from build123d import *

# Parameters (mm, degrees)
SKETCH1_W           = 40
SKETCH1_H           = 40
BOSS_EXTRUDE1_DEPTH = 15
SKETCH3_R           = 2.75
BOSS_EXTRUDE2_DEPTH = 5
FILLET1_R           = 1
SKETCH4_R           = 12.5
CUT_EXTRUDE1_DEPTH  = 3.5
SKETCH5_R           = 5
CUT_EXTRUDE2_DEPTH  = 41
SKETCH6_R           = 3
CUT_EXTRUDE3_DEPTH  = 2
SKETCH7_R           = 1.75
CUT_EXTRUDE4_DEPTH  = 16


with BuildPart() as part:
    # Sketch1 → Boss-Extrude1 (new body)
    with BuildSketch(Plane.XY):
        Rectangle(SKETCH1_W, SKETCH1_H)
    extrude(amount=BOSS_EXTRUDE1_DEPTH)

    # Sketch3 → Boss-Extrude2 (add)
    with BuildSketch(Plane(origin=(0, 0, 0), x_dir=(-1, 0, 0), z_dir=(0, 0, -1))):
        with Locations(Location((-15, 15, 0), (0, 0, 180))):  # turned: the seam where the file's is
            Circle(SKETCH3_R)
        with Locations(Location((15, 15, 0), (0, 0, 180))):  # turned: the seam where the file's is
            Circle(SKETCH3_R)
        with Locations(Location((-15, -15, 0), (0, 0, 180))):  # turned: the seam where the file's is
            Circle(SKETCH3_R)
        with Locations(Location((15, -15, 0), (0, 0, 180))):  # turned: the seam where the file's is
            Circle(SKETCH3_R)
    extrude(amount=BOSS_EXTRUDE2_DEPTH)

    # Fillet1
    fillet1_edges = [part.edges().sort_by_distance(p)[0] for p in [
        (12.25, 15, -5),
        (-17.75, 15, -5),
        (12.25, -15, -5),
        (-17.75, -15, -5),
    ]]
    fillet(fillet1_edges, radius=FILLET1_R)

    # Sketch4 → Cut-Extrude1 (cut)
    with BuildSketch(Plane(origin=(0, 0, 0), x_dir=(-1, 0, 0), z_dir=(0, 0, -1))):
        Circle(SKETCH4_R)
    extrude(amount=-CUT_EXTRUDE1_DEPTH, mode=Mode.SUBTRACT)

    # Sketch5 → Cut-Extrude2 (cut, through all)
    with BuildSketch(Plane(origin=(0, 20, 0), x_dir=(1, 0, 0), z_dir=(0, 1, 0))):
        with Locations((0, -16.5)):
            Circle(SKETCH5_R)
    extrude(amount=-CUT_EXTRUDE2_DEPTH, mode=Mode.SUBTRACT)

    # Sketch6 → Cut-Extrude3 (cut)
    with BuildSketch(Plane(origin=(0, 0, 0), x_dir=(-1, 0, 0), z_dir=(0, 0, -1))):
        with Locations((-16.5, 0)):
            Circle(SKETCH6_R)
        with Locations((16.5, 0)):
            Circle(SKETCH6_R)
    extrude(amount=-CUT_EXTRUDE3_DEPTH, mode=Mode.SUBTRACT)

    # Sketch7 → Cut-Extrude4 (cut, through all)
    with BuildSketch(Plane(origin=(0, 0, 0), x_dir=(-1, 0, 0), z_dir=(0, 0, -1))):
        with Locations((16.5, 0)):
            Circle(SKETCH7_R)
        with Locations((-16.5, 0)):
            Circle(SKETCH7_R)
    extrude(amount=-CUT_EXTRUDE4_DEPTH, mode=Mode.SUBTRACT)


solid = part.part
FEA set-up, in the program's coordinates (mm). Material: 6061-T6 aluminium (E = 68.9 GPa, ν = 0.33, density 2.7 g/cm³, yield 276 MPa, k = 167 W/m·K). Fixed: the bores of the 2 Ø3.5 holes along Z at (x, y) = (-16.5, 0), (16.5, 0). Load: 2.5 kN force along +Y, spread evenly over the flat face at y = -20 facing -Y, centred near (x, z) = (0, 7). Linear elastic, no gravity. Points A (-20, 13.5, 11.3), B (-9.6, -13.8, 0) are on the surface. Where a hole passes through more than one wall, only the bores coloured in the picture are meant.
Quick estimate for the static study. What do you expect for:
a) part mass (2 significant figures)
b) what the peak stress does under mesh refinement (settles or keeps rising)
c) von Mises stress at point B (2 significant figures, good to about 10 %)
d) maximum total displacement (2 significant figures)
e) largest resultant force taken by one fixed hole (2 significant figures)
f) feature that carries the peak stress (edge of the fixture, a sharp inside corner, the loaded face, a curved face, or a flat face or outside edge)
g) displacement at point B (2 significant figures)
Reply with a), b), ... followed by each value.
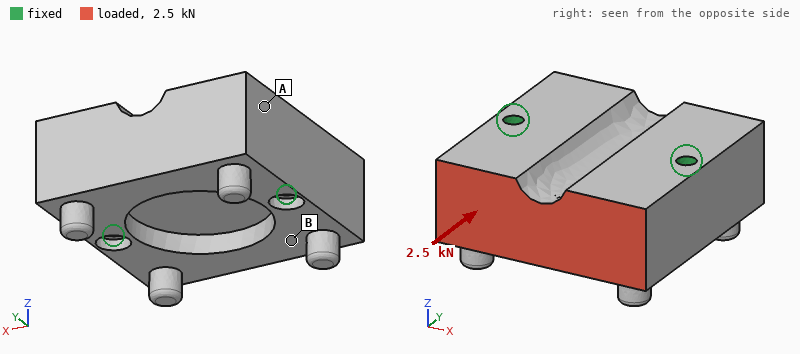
a) 58 g
b) keeps rising
c) 5.9 MPa
d) 3.7 µm
e) 1.3 kN
f) edge of the fixture
g) 2.5 µm
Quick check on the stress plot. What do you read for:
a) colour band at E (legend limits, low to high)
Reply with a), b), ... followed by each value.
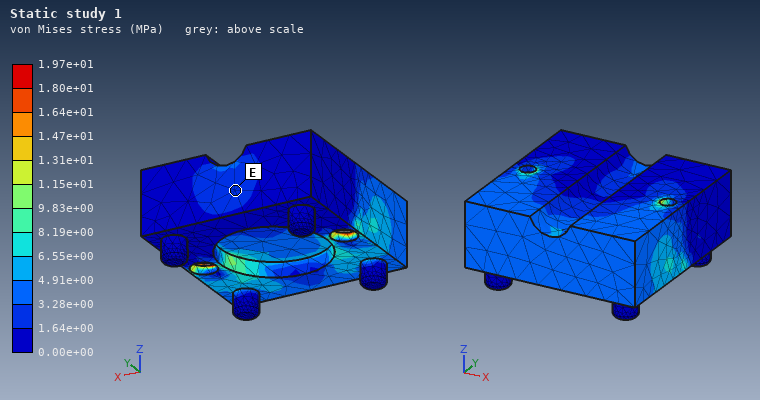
a) 1.64e+00 to 3.28e+00 MPa
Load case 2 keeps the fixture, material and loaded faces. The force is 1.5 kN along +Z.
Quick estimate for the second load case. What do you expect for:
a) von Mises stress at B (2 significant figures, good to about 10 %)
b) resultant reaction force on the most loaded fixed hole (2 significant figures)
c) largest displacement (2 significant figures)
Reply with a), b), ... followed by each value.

a) 9.0 MPa
b) 750 N
c) 19 µm
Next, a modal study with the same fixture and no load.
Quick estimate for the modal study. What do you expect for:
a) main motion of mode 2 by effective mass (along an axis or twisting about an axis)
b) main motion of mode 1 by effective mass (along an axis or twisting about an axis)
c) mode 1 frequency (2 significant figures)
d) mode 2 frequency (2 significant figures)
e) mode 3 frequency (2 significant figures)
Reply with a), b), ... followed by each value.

a) along Z
b) twisting about X
c) 14 kHz
d) 17 kHz
e) 22 kHz
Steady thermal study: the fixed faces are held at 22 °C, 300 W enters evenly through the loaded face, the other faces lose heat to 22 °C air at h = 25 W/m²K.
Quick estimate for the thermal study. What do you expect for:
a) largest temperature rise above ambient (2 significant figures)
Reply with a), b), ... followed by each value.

a) 83 K
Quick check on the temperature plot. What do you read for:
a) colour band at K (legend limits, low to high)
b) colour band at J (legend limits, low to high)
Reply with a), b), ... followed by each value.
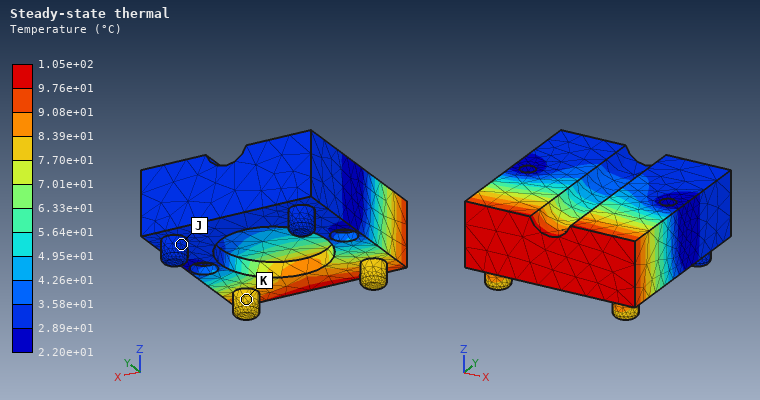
a) 7.70e+01 to 8.39e+01 °C
b) 2.89e+01 to 3.58e+01 °C
